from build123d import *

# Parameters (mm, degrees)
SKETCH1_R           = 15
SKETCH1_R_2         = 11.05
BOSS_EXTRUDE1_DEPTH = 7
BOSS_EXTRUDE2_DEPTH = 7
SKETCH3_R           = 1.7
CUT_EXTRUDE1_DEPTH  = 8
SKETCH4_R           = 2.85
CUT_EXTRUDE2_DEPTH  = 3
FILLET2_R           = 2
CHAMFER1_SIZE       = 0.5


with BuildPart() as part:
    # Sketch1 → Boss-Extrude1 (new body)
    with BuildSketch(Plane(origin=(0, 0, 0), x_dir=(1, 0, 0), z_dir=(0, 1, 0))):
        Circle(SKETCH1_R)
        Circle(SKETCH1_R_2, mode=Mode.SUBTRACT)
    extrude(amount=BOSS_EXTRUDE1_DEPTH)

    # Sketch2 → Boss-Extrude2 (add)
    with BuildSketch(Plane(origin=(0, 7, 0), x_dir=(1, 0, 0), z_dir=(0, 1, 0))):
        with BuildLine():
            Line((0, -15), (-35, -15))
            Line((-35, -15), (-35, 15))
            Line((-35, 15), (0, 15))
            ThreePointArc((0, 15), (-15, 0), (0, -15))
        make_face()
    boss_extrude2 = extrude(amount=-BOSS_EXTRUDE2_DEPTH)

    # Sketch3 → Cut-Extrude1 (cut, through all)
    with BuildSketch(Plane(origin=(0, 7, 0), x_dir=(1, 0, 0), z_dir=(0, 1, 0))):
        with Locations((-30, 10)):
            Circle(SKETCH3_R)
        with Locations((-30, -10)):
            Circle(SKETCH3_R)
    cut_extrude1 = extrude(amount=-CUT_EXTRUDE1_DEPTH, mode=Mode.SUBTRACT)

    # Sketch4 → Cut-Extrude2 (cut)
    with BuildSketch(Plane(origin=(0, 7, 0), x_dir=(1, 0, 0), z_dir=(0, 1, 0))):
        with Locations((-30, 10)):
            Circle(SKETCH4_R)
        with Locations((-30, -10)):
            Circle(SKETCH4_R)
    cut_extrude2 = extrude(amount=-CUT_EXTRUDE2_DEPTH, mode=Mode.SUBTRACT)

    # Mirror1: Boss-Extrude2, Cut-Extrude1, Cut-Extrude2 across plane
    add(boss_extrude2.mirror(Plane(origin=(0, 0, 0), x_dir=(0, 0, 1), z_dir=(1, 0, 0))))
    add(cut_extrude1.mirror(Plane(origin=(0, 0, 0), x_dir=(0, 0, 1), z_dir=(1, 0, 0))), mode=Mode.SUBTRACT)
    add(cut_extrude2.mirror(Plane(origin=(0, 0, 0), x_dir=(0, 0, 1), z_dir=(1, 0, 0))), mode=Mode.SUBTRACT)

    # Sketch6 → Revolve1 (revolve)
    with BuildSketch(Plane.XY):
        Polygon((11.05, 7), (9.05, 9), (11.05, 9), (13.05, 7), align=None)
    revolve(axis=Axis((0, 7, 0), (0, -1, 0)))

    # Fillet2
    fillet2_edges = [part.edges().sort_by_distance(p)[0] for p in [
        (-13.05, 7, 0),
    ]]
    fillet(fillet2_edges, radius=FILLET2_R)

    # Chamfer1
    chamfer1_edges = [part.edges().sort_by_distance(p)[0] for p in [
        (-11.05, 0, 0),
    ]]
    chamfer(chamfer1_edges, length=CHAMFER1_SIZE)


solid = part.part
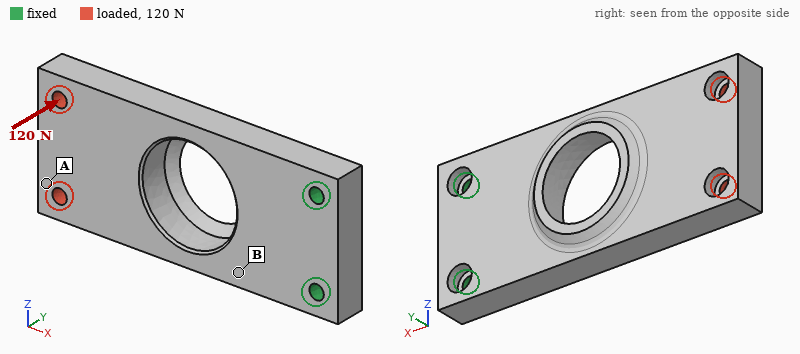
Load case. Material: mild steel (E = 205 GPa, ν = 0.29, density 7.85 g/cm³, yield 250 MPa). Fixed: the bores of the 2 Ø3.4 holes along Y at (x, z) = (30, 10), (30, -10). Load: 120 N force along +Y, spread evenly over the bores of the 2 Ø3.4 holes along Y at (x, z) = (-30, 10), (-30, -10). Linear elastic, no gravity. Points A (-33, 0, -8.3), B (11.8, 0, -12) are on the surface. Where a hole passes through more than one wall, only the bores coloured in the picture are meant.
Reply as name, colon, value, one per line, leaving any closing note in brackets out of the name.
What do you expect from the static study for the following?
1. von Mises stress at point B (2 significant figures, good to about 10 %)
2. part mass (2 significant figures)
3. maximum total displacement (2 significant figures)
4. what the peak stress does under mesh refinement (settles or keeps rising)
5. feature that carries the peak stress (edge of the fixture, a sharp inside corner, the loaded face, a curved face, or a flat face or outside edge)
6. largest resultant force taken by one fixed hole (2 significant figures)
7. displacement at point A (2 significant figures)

von Mises stress at point B: 33 MPa
part mass: 93 g
maximum total displacement: 0.10 mm
what the peak stress does under mesh refinement: keeps rising
feature that carries the peak stress: edge of the fixture
largest resultant force taken by one fixed hole: 64 N
displacement at point A: 0.099 mm
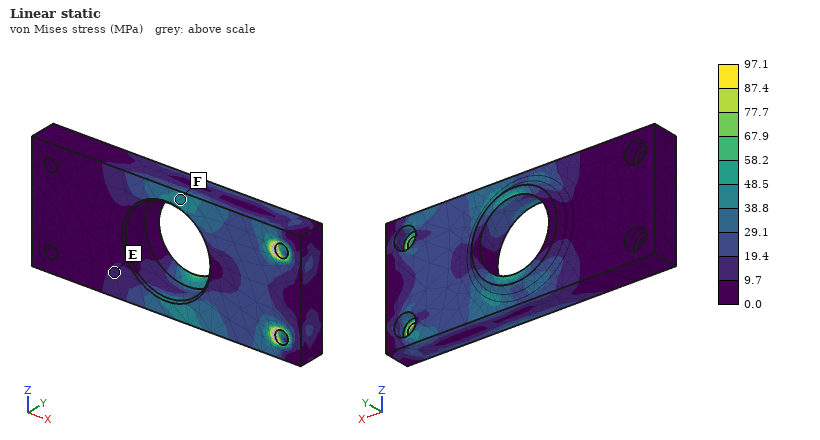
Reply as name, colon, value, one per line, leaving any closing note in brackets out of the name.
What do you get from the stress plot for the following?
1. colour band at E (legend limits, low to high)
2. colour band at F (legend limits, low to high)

colour band at E: 9.7 to 19.4 MPa
colour band at F: 38.8 to 48.5 MPa
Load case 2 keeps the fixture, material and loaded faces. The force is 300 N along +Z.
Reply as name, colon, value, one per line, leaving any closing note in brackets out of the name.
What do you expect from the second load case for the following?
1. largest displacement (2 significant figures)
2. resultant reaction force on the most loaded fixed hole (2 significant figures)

largest displacement: 20 µm
resultant reaction force on the most loaded fixed hole: 850 N
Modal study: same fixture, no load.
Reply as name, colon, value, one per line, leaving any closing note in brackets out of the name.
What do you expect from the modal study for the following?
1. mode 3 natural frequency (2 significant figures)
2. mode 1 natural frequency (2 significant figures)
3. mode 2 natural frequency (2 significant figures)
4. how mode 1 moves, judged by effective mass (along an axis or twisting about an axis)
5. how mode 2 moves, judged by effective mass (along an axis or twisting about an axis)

mode 3 natural frequency: 4700 Hz
mode 1 natural frequency: 1100 Hz
mode 2 natural frequency: 3500 Hz
how mode 1 moves, judged by effective mass: along Y
how mode 2 moves, judged by effective mass: along Z
